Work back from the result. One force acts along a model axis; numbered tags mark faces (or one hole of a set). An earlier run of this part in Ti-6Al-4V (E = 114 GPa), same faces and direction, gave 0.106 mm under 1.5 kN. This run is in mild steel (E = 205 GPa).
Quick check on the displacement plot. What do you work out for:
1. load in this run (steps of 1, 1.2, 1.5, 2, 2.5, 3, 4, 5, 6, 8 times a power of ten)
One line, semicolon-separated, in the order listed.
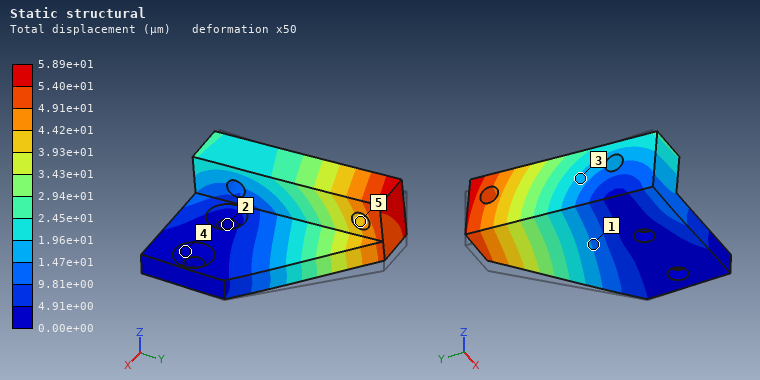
1.5 kN
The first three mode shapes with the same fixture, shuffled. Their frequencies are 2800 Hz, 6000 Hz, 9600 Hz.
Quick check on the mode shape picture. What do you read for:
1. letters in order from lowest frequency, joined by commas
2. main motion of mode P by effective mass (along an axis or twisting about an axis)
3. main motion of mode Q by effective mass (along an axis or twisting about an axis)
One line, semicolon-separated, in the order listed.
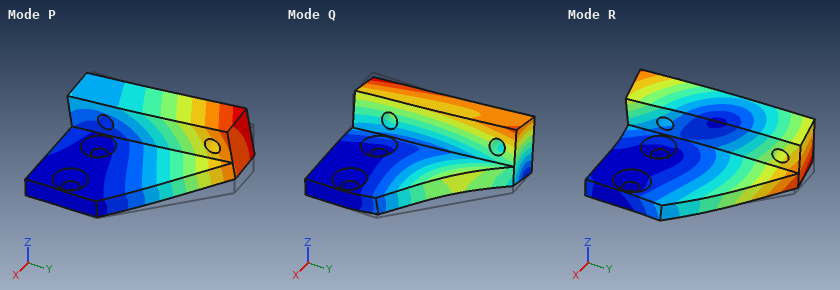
P, Q, R; along Z; along X
